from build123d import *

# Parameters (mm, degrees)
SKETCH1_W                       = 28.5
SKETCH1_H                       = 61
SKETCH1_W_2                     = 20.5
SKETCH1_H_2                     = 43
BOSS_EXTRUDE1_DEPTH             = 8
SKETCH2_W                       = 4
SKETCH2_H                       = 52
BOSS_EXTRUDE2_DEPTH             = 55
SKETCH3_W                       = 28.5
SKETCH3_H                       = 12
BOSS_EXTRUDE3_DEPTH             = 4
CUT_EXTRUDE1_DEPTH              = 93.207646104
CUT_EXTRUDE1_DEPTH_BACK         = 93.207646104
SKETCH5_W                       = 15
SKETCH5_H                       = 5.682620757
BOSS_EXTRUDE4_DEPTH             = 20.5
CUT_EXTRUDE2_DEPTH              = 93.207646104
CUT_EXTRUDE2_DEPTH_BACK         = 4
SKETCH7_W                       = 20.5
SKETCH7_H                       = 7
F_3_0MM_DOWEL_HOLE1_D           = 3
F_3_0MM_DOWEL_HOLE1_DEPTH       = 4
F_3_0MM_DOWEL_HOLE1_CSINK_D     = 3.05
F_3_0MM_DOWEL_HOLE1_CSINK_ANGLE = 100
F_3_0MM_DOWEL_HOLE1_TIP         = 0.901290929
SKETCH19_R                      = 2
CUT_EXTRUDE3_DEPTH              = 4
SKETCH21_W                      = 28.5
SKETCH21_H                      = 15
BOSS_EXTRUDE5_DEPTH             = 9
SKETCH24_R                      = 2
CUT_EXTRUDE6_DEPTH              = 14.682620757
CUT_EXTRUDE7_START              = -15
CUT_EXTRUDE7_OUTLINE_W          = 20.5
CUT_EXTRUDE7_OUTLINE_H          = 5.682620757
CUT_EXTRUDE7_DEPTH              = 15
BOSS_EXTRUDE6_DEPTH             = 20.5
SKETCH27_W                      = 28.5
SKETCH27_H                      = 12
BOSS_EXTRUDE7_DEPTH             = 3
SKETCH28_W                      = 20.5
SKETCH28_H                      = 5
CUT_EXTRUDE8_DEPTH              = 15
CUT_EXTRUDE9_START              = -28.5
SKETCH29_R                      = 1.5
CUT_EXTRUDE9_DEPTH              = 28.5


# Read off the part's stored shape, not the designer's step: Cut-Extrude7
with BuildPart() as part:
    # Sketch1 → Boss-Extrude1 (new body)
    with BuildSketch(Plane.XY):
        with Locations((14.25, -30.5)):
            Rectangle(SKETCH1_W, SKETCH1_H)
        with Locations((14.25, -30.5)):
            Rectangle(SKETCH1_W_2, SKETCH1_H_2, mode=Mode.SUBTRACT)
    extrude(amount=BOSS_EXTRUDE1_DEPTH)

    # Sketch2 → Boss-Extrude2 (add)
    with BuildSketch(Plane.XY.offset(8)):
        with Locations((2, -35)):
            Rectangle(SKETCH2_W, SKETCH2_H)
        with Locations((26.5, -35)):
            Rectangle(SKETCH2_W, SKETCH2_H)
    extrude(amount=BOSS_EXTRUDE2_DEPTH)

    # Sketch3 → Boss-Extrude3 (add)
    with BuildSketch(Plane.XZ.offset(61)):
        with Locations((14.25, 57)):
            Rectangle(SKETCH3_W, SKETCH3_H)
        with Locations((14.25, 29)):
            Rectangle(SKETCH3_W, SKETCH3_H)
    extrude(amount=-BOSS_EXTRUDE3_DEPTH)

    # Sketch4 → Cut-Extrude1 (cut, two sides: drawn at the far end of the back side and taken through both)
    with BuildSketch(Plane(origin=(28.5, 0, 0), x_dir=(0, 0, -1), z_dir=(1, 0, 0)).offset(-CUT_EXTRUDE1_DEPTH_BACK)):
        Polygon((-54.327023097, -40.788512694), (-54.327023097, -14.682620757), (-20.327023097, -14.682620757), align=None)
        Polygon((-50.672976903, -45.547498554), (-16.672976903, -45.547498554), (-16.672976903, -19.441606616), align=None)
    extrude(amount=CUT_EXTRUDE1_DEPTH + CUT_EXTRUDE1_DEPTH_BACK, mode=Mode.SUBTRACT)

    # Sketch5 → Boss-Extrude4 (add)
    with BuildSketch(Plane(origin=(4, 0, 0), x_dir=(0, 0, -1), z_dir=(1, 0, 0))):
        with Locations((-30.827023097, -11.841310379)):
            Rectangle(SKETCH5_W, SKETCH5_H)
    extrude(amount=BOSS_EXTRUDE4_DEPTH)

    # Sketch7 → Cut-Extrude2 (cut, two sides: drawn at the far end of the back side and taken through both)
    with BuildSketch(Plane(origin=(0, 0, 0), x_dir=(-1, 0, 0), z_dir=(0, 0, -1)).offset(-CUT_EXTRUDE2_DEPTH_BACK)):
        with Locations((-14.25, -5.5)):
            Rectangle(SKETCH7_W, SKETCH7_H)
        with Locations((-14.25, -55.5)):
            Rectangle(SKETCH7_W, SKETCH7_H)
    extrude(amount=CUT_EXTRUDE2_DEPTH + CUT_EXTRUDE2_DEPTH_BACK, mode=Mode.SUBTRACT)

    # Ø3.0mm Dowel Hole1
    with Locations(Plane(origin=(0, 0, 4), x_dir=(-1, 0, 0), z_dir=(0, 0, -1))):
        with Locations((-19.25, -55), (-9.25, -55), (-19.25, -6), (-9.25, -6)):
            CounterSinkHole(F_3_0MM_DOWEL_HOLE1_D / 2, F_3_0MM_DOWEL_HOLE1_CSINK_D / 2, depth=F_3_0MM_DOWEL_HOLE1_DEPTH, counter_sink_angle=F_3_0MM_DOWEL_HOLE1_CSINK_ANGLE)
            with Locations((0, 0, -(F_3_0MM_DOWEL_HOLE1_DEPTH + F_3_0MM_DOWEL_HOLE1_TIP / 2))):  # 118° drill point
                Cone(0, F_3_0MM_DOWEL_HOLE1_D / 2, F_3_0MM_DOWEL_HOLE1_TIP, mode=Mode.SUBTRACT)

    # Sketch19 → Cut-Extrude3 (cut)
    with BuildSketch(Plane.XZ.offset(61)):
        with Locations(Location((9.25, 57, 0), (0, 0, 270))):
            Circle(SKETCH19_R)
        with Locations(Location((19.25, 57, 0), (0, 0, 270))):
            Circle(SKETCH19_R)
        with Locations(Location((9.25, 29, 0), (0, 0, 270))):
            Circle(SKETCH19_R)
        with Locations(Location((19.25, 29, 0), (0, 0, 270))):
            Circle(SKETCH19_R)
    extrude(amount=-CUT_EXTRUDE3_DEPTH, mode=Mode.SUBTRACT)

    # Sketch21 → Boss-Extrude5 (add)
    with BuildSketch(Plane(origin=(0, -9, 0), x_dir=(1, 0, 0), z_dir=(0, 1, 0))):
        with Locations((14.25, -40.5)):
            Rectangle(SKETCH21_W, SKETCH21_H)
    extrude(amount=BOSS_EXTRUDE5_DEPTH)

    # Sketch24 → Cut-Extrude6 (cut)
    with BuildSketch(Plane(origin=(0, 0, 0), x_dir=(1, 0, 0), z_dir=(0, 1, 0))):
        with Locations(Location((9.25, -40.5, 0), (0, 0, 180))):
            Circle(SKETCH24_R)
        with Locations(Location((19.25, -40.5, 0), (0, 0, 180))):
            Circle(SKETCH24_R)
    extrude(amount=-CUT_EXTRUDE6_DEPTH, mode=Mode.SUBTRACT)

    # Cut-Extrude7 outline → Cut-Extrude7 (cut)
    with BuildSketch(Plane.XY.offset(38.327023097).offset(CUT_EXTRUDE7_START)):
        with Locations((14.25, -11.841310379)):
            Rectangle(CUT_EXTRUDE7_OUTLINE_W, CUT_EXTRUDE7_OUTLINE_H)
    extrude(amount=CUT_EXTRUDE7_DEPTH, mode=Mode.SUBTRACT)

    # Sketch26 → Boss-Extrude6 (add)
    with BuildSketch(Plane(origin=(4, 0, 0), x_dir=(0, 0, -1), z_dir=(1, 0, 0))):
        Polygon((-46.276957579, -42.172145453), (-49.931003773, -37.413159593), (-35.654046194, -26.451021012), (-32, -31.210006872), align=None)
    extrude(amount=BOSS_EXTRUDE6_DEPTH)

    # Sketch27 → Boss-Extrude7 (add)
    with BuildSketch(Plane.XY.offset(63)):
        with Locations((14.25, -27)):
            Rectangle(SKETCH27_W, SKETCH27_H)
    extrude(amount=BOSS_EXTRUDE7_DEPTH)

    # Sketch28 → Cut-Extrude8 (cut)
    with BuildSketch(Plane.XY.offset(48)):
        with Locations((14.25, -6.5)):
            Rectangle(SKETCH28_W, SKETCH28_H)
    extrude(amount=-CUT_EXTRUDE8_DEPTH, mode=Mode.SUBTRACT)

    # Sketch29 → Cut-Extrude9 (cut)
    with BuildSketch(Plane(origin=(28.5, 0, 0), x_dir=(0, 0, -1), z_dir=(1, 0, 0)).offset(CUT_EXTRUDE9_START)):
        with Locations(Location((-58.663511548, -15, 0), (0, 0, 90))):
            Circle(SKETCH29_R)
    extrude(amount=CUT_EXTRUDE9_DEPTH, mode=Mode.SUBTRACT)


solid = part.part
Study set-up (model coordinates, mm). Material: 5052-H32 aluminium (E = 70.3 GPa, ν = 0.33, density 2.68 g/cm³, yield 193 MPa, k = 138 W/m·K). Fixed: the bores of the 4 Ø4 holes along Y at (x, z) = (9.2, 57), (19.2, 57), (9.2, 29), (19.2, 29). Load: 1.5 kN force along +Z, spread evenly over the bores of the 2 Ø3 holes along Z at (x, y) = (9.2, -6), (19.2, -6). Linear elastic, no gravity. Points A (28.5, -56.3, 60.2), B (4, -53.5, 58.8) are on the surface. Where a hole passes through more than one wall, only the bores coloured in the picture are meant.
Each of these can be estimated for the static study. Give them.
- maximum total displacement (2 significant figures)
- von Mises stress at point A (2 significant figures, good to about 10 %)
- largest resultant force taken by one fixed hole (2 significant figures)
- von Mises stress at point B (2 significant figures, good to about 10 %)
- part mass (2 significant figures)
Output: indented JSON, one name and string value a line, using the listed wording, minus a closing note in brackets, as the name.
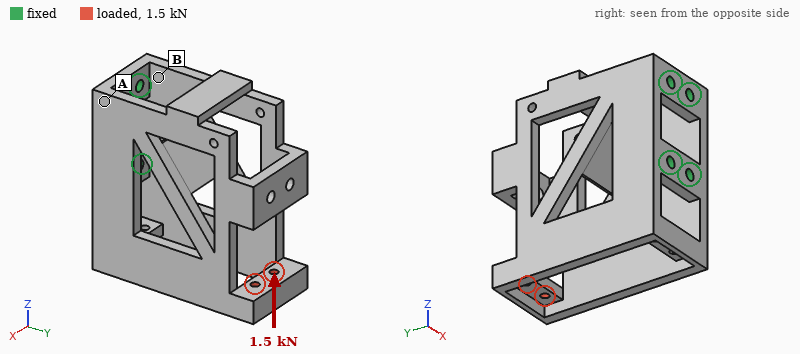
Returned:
{
  "maximum total displacement": "0.25 mm",
  "von Mises stress at point A": "31 MPa",
  "largest resultant force taken by one fixed hole": "1.4 kN",
  "von Mises stress at point B": "73 MPa",
  "part mass": "76 g"
}
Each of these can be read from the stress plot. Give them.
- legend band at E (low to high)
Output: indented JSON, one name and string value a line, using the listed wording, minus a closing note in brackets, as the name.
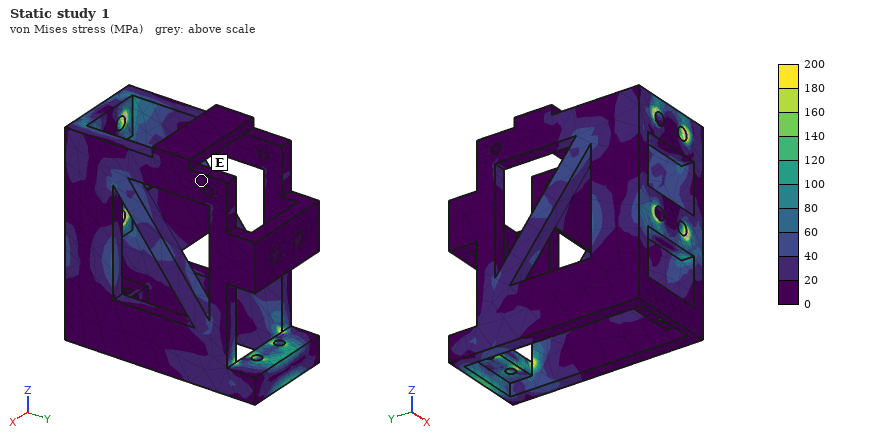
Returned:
{
  "legend band at E": "0 to 20 MPa"
}
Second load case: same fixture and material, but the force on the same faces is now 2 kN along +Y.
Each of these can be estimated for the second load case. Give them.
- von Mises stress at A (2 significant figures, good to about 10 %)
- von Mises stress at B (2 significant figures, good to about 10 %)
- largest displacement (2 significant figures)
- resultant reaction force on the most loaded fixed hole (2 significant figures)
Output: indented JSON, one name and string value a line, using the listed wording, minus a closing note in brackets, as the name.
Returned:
{
  "von Mises stress at A": "20 MPa",
  "von Mises stress at B": "39 MPa",
  "largest displacement": "0.21 mm",
  "resultant reaction force on the most loaded fixed hole": "1.7 kN"
}
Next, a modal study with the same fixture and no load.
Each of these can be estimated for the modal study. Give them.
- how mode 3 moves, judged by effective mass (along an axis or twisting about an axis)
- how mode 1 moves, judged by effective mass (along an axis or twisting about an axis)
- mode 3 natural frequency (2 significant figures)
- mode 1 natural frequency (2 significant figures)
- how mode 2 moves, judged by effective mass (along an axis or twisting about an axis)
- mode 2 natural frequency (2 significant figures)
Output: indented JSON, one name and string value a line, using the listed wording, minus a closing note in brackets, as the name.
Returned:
{
  "how mode 3 moves, judged by effective mass": "twisting about Y",
  "how mode 1 moves, judged by effective mass": "along X",
  "mode 3 natural frequency": "2700 Hz",
  "mode 1 natural frequency": "1300 Hz",
  "how mode 2 moves, judged by effective mass": "along Z",
  "mode 2 natural frequency": "2600 Hz"
}
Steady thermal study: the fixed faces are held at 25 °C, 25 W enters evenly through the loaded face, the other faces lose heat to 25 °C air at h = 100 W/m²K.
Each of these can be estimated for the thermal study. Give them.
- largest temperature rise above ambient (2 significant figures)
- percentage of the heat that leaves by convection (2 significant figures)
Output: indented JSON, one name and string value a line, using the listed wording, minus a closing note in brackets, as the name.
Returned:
{
  "largest temperature rise above ambient": "59 K",
  "percentage of the heat that leaves by convection": "72 %"
}
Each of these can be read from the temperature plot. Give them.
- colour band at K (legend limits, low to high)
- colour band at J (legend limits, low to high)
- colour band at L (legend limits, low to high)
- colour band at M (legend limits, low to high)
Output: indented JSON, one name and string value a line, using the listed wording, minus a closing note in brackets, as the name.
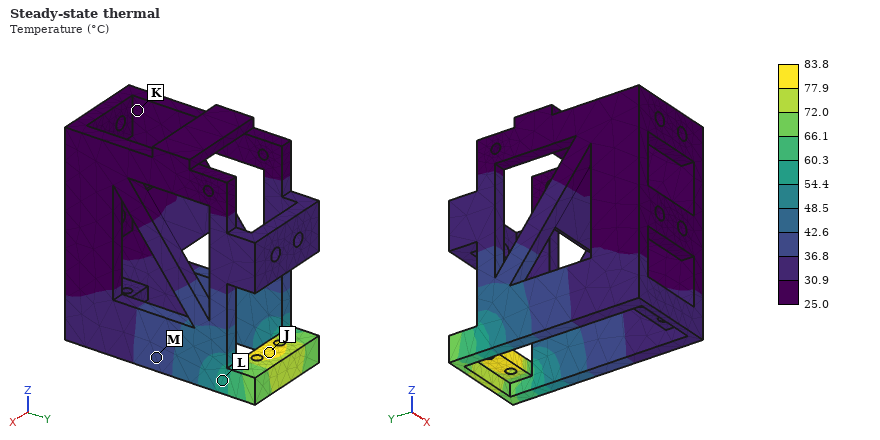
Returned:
{
  "colour band at K": "25.0 to 30.9 °C",
  "colour band at J": "77.9 to 83.8 °C",
  "colour band at L": "54.4 to 60.3 °C",
  "colour band at M": "36.8 to 42.6 °C"
}
